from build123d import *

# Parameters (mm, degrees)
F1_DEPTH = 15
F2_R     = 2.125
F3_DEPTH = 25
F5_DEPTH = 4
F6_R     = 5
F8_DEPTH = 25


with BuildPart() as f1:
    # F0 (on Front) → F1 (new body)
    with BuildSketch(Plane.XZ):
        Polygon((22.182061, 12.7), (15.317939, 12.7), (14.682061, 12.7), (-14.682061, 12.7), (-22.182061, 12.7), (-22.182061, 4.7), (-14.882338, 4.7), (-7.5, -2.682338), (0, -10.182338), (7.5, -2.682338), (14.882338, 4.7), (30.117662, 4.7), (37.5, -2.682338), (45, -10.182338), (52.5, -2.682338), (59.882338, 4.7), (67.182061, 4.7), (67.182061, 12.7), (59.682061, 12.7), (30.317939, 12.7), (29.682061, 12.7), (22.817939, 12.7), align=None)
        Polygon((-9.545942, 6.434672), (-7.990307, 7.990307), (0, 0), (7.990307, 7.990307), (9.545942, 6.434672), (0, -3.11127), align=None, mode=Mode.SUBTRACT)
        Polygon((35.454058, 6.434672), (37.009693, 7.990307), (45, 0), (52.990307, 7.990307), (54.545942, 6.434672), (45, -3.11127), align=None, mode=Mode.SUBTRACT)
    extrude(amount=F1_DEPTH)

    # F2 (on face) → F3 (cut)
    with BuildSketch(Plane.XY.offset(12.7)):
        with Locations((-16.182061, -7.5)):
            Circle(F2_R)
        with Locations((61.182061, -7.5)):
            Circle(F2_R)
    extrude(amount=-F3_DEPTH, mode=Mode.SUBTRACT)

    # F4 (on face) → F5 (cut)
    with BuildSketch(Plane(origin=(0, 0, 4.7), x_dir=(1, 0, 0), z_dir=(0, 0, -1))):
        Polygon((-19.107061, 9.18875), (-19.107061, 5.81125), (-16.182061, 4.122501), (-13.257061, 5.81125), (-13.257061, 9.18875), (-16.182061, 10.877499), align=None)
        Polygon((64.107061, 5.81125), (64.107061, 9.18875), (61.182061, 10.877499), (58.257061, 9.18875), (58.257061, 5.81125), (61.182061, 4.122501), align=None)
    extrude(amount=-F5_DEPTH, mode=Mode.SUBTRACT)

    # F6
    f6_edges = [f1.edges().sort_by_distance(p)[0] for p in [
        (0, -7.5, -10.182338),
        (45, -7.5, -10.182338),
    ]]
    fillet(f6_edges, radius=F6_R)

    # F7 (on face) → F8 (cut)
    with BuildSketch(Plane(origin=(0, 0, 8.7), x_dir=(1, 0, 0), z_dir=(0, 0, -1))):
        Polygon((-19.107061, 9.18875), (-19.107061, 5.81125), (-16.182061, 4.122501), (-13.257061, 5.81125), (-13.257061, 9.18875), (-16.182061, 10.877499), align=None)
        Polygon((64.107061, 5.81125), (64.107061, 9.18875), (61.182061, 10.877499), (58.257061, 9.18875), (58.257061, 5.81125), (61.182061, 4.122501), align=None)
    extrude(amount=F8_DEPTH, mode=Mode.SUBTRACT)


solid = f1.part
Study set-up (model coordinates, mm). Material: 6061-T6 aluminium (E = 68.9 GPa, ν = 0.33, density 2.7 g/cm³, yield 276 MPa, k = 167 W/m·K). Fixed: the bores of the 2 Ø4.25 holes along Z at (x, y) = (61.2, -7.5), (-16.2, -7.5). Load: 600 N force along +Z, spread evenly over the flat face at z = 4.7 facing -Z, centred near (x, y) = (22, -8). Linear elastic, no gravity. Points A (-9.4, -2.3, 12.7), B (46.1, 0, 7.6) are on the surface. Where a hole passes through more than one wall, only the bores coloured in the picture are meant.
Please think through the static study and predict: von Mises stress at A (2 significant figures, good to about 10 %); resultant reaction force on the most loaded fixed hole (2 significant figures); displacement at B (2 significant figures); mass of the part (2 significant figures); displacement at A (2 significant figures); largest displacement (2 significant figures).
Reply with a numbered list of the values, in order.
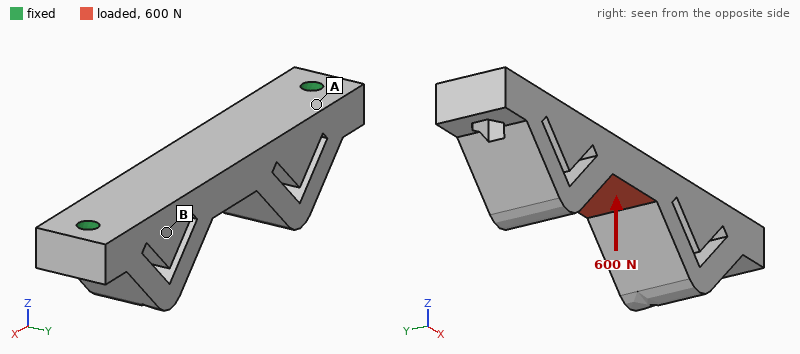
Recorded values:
1. 24 MPa
2. 460 N
3. 23 µm
4. 41 g
5. 8.4 µm
6. 54 µm
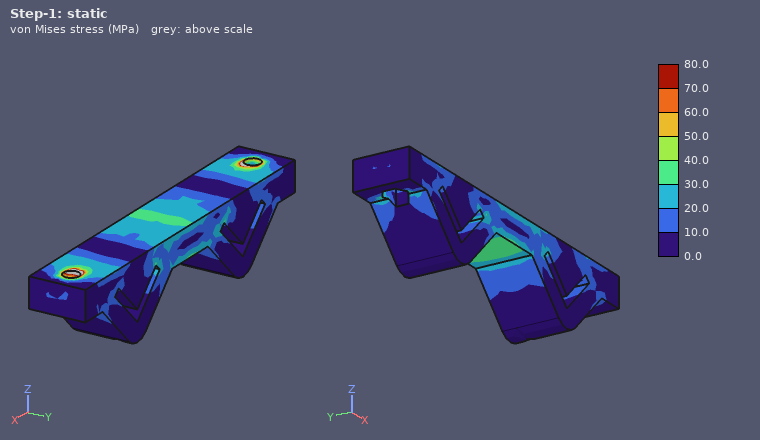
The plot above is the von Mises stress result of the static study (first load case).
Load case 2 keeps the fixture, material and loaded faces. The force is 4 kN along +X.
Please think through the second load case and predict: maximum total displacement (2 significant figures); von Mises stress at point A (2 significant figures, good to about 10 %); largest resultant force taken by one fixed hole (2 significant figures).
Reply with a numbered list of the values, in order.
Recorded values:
1. 17 µm
2. 29 MPa
3. 2.0 kN
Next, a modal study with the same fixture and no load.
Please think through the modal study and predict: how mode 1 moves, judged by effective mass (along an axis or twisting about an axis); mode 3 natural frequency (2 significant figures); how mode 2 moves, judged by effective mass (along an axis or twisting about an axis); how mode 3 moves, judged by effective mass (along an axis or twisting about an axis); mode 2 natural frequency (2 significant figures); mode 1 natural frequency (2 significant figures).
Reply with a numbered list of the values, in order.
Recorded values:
1. along Z
2. 9500 Hz
3. along Y
4. twisting about X
5. 5800 Hz
6. 4200 Hz
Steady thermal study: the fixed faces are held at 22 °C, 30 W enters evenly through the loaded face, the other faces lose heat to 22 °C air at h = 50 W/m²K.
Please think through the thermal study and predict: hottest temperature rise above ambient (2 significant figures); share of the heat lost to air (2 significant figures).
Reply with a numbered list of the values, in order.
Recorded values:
1. 24 K
2. 12 %
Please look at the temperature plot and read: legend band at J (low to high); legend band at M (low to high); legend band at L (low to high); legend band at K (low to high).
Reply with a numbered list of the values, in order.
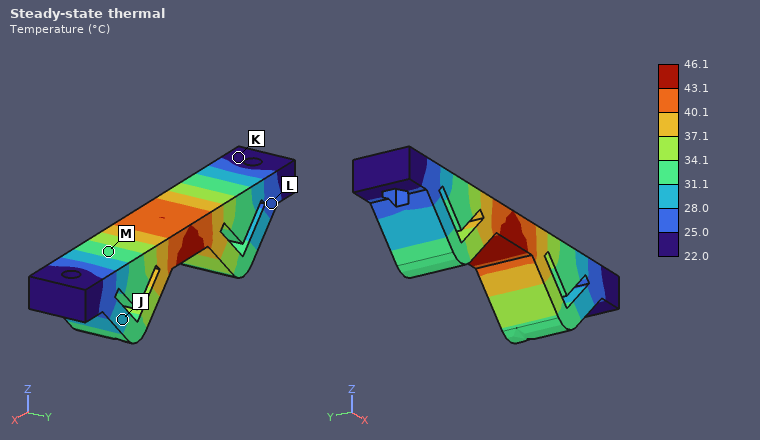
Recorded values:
1. 28.0 to 31.1 °C
2. 31.1 to 34.1 °C
3. 25.0 to 28.0 °C
4. 22.0 to 25.0 °C
